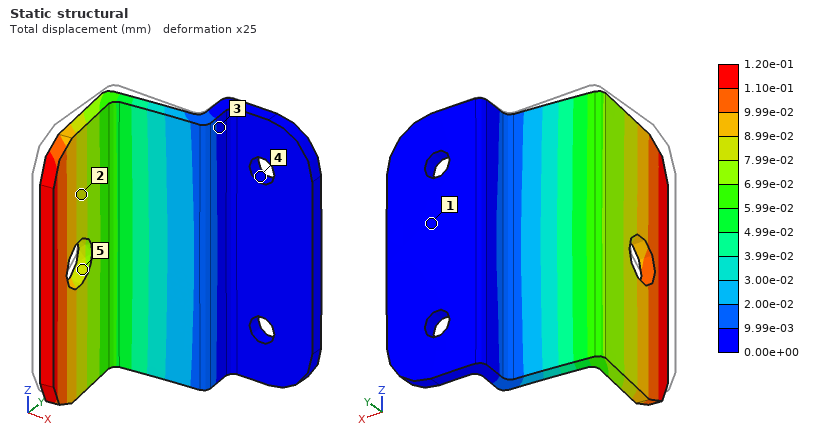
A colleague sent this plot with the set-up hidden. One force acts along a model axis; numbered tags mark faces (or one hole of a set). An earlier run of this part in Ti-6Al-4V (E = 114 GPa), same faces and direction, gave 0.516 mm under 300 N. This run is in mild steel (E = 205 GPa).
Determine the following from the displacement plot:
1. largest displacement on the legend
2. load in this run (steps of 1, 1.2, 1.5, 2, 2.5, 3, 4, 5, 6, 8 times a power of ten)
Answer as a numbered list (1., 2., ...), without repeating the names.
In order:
1. 1.20e-01 mm
2. 120 N
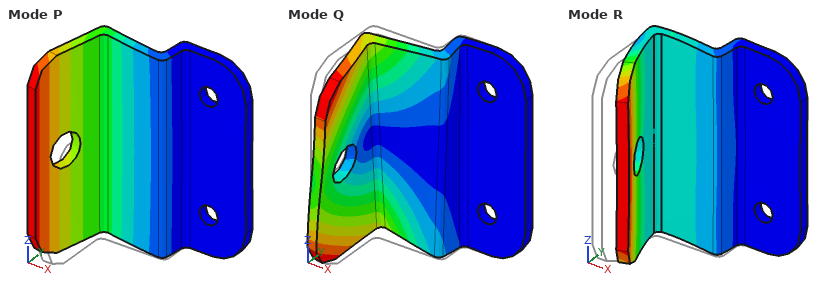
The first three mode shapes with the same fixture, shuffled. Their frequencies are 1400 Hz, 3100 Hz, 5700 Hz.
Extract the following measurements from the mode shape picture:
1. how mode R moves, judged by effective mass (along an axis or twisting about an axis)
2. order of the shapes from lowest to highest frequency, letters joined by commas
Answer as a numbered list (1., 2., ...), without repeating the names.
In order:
1. along Y
2. P, Q, R
